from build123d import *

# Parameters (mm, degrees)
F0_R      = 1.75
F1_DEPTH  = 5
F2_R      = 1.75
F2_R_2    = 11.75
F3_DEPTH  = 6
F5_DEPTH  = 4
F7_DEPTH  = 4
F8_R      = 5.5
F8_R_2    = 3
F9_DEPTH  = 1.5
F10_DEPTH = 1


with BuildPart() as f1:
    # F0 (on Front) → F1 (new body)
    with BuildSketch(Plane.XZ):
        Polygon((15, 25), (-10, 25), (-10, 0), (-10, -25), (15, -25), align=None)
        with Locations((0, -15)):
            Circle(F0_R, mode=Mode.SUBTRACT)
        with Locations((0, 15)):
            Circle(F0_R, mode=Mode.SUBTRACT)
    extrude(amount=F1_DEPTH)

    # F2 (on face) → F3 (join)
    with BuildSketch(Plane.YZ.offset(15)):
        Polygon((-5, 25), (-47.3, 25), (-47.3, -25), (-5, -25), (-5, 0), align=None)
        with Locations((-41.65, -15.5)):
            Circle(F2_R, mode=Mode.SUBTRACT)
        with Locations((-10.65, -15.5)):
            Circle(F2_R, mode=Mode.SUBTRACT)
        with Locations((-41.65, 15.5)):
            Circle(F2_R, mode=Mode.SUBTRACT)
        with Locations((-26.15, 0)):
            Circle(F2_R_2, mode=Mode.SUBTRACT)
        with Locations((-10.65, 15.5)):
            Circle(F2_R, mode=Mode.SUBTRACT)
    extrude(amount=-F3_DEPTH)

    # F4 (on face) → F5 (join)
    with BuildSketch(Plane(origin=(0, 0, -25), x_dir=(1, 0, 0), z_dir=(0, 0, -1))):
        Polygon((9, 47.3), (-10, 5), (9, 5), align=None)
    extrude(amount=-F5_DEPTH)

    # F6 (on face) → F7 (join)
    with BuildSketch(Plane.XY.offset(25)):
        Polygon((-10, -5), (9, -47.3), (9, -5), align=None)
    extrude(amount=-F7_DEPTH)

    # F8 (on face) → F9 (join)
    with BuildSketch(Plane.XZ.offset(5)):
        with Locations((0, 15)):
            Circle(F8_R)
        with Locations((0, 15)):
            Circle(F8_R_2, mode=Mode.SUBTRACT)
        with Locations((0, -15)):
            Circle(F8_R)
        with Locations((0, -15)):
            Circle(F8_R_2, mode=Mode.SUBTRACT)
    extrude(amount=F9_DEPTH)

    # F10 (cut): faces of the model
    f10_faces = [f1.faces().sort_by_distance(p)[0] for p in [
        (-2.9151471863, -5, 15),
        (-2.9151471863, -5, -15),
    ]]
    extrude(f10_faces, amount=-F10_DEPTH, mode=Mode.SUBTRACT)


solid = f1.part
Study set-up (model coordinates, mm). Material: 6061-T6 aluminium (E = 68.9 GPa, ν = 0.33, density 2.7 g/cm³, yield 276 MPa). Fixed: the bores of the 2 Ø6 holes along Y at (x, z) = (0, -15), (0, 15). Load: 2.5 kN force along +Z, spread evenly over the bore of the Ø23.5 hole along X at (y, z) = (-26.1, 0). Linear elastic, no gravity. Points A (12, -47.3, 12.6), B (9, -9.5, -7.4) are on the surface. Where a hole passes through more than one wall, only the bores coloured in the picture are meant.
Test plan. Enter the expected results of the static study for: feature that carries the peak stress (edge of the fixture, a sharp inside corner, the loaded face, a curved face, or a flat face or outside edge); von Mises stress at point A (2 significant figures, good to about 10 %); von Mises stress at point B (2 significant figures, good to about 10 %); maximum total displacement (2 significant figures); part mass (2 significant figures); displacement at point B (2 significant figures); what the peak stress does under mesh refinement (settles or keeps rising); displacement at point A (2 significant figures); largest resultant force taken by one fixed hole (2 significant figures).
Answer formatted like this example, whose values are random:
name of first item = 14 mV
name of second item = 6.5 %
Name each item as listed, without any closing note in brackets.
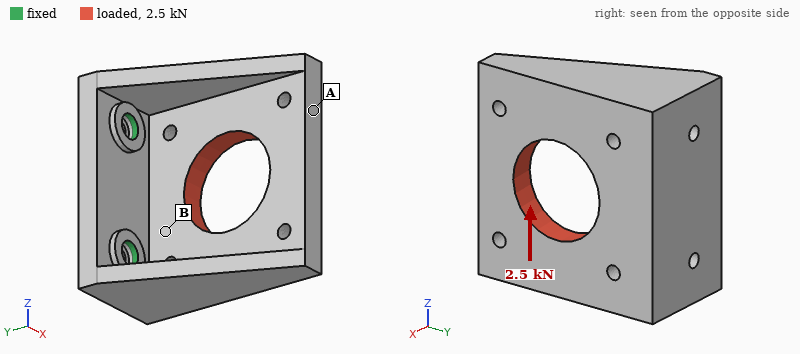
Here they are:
feature that carries the peak stress = edge of the fixture
von Mises stress at point A = 24 MPa
von Mises stress at point B = 55 MPa
maximum total displacement = 0.17 mm
part mass = 52 g
displacement at point B = 0.026 mm
what the peak stress does under mesh refinement = keeps rising
displacement at point A = 0.14 mm
largest resultant force taken by one fixed hole = 2.1 kN
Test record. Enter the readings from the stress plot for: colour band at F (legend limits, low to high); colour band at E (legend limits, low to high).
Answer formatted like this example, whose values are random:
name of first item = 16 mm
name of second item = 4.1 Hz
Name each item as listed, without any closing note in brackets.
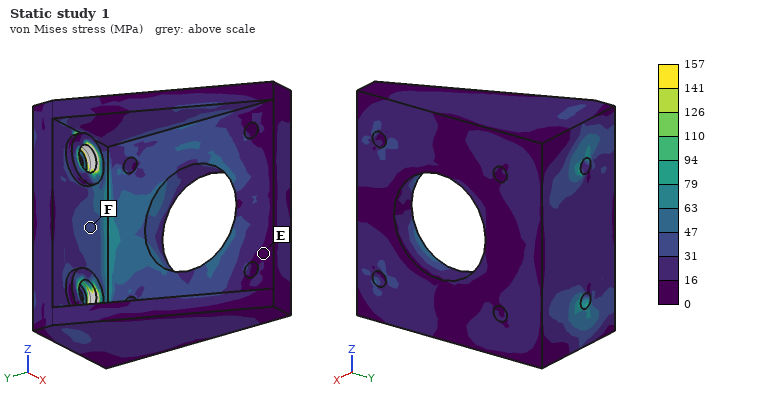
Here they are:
colour band at F = 31 to 47 MPa
colour band at E = 0 to 16 MPa
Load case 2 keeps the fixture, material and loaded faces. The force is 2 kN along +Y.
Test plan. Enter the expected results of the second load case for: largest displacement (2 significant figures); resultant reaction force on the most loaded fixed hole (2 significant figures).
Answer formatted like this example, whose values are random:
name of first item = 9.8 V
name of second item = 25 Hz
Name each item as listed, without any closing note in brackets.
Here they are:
largest displacement = 0.20 mm
resultant reaction force on the most loaded fixed hole = 1.0 kN
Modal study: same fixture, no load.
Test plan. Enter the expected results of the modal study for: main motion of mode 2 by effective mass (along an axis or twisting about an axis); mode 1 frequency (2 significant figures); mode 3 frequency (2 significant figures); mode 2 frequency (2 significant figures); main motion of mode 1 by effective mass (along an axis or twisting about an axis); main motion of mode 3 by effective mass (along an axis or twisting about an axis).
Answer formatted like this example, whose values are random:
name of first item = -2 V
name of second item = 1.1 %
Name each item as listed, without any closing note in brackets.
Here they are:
main motion of mode 2 by effective mass = along Z
mode 1 frequency = 2200 Hz
mode 3 frequency = 7800 Hz
mode 2 frequency = 3600 Hz
main motion of mode 1 by effective mass = along X
main motion of mode 3 by effective mass = along Z
